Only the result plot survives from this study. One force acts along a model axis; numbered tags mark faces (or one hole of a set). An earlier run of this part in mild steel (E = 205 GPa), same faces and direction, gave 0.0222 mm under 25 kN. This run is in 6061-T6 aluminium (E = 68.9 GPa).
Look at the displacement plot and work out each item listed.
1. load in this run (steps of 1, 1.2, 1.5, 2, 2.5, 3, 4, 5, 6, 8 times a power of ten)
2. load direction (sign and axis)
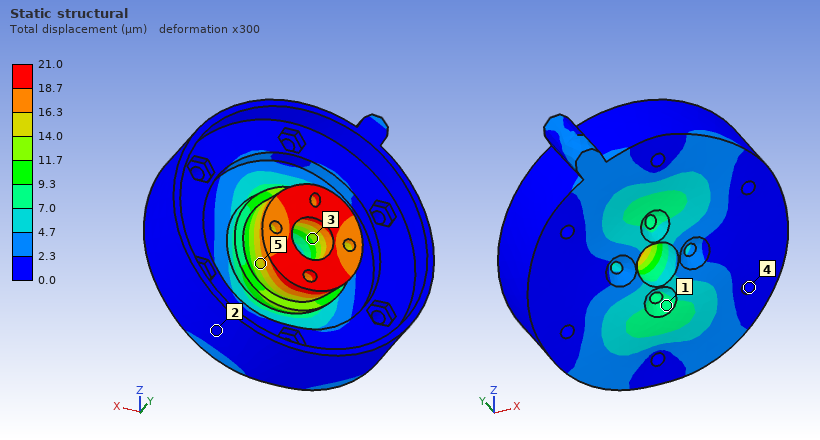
8 kN
-Z
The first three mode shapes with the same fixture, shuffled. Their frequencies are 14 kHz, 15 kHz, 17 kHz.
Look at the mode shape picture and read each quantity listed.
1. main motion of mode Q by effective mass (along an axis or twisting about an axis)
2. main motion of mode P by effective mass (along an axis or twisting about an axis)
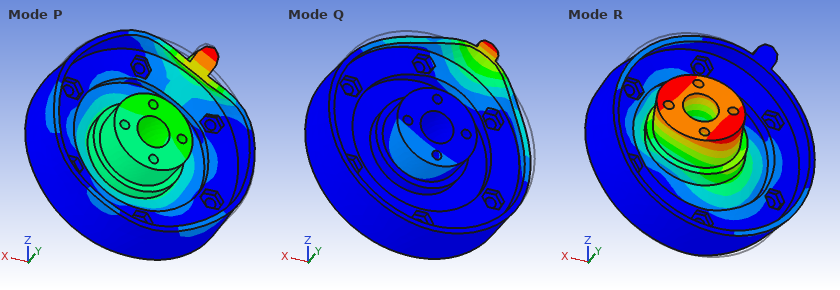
along Y
along Y
